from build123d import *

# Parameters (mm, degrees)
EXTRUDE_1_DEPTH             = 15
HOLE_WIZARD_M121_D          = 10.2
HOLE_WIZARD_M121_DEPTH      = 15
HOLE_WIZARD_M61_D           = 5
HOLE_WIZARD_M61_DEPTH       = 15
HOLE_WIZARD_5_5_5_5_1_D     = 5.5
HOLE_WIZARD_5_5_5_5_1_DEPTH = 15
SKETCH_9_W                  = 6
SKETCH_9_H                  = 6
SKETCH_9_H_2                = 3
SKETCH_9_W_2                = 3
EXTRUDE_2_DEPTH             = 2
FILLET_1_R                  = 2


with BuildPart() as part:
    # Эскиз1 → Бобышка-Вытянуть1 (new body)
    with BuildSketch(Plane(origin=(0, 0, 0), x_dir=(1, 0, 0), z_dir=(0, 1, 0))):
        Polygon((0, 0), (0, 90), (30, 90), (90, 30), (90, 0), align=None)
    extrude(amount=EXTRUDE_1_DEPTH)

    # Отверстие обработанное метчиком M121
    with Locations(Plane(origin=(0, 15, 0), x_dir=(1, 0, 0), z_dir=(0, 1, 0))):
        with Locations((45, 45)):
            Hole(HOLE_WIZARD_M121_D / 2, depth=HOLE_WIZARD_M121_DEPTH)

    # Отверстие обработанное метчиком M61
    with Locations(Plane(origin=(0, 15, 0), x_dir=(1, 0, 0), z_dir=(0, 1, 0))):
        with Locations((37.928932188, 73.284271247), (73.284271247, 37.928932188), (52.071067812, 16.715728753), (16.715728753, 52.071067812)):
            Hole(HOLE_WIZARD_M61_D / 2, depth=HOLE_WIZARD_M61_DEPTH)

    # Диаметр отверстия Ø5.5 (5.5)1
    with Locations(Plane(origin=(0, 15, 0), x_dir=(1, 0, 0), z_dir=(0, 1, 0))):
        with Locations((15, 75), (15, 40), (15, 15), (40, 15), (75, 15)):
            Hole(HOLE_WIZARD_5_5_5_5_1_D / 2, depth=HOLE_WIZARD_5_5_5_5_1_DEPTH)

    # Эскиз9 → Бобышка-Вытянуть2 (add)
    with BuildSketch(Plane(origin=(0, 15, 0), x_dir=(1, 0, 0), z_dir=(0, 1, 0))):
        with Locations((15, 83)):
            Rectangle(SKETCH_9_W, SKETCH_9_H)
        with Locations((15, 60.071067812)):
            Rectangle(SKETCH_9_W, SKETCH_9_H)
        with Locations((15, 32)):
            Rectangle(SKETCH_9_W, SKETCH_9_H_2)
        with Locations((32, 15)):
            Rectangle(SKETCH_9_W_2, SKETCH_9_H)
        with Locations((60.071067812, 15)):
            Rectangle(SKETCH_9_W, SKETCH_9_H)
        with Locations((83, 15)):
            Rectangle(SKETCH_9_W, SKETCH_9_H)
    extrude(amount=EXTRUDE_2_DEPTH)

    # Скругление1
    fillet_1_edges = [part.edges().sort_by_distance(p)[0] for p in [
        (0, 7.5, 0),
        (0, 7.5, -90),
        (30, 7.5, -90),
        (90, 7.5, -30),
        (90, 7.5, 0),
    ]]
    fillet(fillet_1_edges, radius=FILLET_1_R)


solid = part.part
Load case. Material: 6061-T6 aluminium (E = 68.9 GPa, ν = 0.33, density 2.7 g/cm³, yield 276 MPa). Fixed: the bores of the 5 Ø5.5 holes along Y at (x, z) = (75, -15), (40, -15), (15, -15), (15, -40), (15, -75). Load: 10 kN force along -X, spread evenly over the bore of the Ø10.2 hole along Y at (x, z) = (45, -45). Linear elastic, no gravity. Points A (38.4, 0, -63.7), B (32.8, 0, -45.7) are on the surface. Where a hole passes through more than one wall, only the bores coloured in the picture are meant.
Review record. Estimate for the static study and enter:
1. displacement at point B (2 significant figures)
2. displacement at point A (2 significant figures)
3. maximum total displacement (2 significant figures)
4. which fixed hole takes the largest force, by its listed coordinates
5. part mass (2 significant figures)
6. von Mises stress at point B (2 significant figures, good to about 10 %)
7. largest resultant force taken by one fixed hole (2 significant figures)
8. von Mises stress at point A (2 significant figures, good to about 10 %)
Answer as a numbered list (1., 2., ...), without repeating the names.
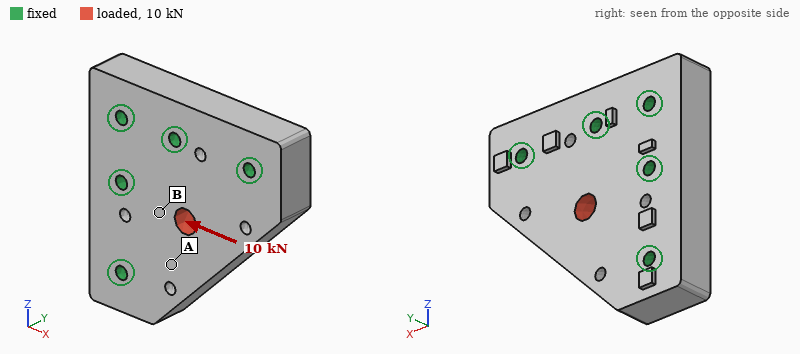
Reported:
1. 4.4 µm
2. 3.1 µm
3. 8.8 µm
4. (15, -40)
5. 240 g
6. 19 MPa
7. 4.0 kN
8. 6.7 MPa
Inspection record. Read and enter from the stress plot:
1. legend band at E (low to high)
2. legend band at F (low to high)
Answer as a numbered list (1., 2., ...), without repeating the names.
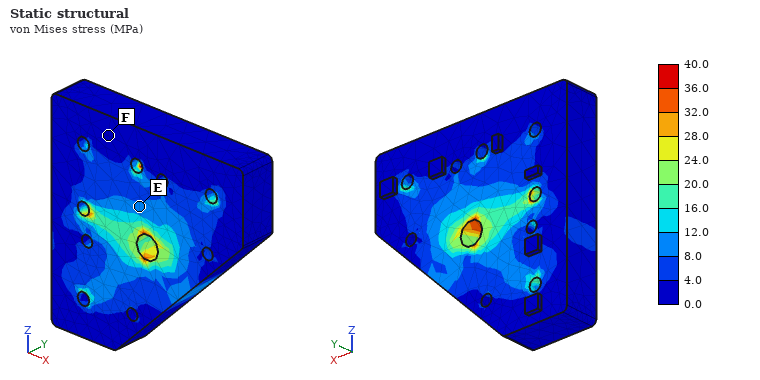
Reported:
1. 8.0 to 12.0 MPa
2. 0.0 to 4.0 MPa
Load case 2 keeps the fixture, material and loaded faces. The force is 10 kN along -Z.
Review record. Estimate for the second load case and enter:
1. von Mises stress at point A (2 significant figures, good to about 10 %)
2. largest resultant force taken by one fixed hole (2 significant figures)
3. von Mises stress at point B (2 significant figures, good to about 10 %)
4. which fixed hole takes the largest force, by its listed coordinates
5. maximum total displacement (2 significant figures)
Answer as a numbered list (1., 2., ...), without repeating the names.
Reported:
1. 9.3 MPa
2. 4.0 kN
3. 11 MPa
4. (40, -15)
5. 8.7 µm
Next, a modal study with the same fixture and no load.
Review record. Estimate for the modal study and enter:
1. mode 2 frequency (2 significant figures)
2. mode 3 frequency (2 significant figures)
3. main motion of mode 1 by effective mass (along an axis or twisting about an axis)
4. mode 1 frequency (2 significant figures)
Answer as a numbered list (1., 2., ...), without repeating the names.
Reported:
1. 18 kHz
2. 23 kHz
3. along Y
4. 9300 Hz
